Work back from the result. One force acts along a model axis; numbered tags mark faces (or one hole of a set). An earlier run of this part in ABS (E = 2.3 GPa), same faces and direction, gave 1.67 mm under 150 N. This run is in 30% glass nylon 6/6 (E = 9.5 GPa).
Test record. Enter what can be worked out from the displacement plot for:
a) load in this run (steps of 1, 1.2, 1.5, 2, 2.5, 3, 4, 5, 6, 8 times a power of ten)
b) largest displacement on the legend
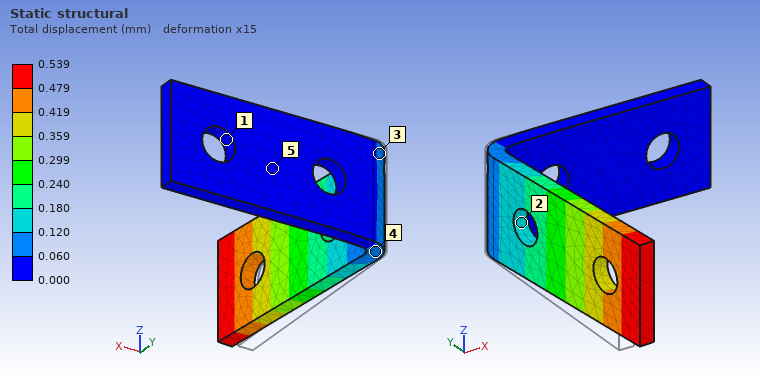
200 N
0.539 mm
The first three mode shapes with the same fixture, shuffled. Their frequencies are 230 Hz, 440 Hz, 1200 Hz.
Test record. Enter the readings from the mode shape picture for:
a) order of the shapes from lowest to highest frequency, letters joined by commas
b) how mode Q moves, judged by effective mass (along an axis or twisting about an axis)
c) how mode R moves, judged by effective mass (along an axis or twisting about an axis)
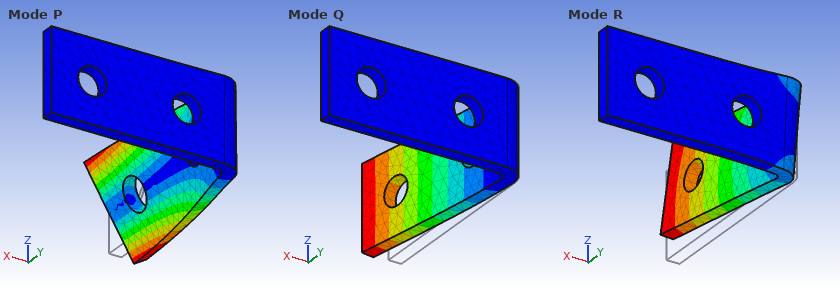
Q, R, P
along X
along Z
